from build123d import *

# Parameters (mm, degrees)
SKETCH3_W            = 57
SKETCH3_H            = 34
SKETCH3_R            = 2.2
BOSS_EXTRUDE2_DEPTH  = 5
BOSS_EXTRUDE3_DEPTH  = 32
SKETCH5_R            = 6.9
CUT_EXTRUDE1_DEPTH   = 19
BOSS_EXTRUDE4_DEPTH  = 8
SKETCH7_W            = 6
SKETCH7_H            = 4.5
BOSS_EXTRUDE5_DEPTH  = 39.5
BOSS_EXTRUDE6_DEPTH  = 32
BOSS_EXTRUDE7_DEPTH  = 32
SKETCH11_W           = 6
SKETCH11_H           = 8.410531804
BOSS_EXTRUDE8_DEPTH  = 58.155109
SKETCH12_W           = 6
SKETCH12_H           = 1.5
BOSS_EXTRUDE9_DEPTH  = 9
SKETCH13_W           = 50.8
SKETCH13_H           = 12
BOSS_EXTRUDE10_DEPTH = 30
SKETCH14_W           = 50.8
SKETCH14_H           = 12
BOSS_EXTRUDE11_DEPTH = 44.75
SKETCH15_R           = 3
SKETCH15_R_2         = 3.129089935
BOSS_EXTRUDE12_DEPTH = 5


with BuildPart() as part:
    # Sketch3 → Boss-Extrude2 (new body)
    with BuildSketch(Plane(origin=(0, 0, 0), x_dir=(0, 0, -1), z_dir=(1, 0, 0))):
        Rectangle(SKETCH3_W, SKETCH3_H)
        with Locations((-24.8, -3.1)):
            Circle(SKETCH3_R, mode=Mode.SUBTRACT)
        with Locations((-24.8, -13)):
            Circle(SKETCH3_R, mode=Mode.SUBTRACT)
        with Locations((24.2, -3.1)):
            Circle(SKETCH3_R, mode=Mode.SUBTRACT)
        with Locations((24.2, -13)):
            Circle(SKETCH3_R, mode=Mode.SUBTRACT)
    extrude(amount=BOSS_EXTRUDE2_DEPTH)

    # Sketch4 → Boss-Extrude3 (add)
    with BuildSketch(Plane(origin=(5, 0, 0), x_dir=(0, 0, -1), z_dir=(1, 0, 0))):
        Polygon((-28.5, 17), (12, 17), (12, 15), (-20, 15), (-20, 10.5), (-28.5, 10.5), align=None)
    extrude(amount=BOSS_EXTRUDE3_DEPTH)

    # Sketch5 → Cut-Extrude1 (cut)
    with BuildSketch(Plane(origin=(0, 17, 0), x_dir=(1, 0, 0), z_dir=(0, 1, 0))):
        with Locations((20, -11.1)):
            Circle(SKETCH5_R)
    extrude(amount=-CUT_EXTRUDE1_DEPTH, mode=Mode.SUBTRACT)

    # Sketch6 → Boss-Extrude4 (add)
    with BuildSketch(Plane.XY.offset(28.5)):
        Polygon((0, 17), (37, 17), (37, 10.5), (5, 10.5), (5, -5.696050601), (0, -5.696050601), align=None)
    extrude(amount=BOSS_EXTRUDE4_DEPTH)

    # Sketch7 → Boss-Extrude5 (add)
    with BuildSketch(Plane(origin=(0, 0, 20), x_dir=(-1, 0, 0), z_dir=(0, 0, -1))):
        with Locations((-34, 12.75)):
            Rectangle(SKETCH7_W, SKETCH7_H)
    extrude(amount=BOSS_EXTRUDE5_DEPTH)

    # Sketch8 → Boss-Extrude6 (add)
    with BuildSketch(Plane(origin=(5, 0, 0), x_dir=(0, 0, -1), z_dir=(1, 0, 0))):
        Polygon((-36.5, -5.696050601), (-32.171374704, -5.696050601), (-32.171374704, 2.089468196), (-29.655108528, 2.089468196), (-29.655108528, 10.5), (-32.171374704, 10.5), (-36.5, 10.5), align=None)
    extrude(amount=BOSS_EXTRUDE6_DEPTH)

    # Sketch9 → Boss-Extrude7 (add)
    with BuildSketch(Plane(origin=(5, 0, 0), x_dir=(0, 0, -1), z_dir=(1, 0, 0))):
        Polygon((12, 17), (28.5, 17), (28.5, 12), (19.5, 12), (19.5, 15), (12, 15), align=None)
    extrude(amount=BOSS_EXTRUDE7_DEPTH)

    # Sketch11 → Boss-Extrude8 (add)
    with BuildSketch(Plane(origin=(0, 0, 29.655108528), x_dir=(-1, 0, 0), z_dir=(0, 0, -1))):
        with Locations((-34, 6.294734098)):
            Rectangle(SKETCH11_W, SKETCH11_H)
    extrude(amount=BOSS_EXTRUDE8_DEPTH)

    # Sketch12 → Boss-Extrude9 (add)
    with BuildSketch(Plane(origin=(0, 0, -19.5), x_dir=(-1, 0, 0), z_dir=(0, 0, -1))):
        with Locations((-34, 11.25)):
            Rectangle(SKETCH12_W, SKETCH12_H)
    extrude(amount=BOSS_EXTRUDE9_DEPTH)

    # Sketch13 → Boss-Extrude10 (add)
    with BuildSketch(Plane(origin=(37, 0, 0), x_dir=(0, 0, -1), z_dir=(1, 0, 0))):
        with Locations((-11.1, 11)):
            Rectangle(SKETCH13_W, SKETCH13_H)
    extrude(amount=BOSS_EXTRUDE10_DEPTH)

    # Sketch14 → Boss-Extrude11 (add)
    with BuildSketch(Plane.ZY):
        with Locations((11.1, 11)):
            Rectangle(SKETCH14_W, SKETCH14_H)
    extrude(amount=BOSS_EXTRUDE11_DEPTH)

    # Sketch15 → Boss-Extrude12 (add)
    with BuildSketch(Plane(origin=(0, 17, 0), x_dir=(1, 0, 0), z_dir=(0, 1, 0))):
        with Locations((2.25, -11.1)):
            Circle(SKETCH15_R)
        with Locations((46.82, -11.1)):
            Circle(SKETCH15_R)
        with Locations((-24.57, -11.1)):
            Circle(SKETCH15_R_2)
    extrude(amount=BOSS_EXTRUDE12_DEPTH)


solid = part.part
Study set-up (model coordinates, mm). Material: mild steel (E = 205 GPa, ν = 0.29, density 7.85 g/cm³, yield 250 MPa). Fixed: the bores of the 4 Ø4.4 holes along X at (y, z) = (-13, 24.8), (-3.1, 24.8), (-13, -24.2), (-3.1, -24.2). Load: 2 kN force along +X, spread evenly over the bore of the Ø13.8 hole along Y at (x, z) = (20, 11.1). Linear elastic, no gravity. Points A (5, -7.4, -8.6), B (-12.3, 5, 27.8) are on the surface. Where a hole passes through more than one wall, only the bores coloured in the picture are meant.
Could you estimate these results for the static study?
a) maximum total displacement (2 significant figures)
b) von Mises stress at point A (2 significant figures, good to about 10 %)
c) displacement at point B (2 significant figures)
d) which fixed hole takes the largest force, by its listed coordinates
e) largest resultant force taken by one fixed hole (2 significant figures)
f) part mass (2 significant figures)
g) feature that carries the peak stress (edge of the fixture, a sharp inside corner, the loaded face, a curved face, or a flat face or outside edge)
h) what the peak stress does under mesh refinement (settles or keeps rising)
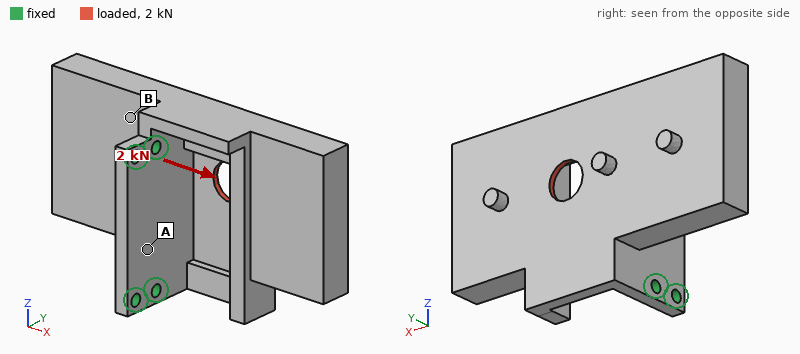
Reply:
0.17 mm
35 MPa
0.040 mm
(-3.1, 24.8)
2.0 kN
550 g
edge of the fixture
keeps rising
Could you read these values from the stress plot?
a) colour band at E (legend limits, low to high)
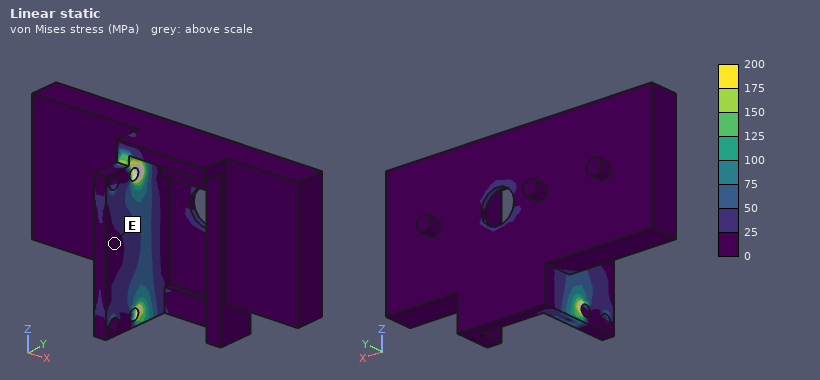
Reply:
0 to 25 MPa
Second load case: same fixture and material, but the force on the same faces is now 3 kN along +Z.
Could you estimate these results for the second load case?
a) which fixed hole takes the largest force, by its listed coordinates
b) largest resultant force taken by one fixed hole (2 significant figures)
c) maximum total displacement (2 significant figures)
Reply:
(-3.1, 24.8)
2.1 kN
59 µm
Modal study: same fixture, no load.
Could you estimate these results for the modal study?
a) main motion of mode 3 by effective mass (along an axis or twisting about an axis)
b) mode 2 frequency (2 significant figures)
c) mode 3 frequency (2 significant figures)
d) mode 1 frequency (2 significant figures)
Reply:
along Y
1700 Hz
2100 Hz
640 Hz
